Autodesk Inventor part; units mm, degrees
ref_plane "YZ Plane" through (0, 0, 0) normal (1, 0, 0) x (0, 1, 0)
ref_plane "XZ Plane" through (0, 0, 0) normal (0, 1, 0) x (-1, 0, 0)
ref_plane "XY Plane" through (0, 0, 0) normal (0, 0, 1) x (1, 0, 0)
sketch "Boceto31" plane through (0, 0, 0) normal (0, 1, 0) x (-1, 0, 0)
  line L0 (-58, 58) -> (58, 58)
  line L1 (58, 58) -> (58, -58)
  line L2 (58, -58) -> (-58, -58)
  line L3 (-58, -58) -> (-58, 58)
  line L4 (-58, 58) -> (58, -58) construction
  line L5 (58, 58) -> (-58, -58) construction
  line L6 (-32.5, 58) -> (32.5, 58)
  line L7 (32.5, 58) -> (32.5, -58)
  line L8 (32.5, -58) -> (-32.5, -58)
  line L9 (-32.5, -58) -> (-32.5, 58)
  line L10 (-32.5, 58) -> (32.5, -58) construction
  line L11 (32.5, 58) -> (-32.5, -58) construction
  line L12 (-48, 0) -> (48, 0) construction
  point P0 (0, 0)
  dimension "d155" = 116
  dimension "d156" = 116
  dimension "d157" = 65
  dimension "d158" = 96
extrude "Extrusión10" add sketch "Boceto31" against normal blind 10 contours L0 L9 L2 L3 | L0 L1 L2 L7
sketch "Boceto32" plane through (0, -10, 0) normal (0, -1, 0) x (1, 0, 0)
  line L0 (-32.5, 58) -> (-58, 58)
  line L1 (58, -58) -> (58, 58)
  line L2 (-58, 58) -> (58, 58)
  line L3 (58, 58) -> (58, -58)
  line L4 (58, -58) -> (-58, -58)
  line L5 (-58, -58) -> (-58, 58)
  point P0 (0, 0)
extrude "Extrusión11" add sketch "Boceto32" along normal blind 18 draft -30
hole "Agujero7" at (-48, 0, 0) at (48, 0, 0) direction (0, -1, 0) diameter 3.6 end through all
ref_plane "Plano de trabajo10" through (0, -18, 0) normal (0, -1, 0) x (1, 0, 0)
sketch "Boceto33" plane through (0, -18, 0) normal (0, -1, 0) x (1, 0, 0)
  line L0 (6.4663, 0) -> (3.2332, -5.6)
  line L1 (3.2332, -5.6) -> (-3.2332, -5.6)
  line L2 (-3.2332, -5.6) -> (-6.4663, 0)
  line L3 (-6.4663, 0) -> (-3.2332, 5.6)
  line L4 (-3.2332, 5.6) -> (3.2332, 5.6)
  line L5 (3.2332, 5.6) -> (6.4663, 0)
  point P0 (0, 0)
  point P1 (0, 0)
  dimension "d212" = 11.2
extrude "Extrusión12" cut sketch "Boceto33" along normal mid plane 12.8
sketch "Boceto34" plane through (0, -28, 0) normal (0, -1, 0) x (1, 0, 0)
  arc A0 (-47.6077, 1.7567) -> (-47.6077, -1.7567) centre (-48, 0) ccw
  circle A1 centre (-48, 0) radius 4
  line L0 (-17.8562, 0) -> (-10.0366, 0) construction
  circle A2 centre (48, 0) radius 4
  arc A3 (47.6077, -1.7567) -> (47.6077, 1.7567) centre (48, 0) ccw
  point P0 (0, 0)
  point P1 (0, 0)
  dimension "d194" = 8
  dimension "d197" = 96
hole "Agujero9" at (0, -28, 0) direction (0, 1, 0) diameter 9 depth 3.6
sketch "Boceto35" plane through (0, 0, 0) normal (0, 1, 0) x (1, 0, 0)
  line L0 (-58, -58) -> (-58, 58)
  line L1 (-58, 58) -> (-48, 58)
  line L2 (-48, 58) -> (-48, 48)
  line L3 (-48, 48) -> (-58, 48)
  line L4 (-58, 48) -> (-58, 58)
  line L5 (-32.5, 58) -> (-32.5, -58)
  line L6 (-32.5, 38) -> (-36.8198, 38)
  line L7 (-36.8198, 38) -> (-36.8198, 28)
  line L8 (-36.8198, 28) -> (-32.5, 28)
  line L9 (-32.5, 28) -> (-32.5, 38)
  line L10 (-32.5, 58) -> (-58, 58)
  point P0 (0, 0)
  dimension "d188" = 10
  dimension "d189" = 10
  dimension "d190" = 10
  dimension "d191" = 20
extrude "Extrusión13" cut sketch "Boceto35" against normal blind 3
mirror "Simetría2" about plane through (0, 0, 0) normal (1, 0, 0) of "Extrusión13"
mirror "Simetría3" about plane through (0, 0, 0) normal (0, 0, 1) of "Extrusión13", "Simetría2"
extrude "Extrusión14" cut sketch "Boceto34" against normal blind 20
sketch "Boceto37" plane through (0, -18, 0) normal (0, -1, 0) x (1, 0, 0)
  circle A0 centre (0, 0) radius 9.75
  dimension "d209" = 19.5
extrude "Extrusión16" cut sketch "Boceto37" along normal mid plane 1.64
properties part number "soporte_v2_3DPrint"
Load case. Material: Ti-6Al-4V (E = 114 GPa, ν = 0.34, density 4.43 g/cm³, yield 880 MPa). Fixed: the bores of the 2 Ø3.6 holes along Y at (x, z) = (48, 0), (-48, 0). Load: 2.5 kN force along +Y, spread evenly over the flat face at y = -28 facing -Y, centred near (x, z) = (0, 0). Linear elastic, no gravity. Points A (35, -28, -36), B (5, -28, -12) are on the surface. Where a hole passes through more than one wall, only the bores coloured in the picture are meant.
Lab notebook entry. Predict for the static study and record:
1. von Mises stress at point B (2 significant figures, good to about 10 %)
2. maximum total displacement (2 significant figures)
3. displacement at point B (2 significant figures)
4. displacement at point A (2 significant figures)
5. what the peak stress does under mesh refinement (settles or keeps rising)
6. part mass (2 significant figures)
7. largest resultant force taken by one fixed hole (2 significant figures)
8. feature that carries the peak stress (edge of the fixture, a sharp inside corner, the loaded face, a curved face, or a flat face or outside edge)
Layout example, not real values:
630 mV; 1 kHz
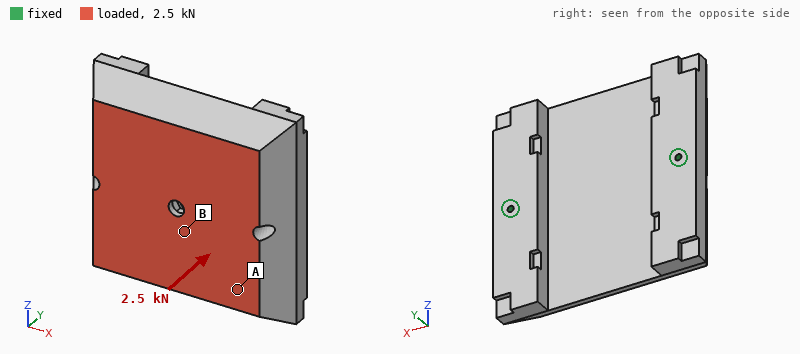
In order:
3.8 MPa; 5.8 µm; 3.9 µm; 3.4 µm; keeps rising; 1.1 kg; 1.6 kN; edge of the fixture
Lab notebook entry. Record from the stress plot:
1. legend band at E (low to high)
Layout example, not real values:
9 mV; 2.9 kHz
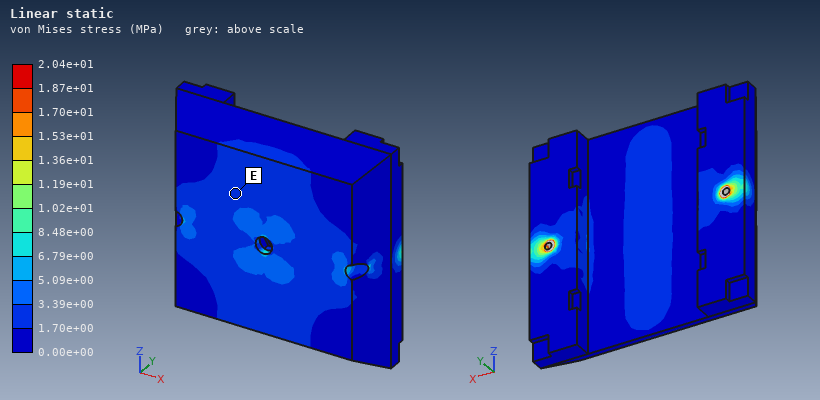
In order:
1.70e+00 to 3.39e+00 MPa
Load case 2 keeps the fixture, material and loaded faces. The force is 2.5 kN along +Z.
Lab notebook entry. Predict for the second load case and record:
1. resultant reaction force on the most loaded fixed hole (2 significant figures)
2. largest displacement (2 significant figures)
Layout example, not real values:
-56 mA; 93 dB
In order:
1.3 kN; 79 µm
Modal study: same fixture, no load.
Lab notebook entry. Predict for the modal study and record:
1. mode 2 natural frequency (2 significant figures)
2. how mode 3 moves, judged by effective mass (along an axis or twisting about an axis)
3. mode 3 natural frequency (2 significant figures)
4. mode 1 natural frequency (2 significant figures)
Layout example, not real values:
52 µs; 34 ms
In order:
3700 Hz; along Y; 4100 Hz; 920 Hz
